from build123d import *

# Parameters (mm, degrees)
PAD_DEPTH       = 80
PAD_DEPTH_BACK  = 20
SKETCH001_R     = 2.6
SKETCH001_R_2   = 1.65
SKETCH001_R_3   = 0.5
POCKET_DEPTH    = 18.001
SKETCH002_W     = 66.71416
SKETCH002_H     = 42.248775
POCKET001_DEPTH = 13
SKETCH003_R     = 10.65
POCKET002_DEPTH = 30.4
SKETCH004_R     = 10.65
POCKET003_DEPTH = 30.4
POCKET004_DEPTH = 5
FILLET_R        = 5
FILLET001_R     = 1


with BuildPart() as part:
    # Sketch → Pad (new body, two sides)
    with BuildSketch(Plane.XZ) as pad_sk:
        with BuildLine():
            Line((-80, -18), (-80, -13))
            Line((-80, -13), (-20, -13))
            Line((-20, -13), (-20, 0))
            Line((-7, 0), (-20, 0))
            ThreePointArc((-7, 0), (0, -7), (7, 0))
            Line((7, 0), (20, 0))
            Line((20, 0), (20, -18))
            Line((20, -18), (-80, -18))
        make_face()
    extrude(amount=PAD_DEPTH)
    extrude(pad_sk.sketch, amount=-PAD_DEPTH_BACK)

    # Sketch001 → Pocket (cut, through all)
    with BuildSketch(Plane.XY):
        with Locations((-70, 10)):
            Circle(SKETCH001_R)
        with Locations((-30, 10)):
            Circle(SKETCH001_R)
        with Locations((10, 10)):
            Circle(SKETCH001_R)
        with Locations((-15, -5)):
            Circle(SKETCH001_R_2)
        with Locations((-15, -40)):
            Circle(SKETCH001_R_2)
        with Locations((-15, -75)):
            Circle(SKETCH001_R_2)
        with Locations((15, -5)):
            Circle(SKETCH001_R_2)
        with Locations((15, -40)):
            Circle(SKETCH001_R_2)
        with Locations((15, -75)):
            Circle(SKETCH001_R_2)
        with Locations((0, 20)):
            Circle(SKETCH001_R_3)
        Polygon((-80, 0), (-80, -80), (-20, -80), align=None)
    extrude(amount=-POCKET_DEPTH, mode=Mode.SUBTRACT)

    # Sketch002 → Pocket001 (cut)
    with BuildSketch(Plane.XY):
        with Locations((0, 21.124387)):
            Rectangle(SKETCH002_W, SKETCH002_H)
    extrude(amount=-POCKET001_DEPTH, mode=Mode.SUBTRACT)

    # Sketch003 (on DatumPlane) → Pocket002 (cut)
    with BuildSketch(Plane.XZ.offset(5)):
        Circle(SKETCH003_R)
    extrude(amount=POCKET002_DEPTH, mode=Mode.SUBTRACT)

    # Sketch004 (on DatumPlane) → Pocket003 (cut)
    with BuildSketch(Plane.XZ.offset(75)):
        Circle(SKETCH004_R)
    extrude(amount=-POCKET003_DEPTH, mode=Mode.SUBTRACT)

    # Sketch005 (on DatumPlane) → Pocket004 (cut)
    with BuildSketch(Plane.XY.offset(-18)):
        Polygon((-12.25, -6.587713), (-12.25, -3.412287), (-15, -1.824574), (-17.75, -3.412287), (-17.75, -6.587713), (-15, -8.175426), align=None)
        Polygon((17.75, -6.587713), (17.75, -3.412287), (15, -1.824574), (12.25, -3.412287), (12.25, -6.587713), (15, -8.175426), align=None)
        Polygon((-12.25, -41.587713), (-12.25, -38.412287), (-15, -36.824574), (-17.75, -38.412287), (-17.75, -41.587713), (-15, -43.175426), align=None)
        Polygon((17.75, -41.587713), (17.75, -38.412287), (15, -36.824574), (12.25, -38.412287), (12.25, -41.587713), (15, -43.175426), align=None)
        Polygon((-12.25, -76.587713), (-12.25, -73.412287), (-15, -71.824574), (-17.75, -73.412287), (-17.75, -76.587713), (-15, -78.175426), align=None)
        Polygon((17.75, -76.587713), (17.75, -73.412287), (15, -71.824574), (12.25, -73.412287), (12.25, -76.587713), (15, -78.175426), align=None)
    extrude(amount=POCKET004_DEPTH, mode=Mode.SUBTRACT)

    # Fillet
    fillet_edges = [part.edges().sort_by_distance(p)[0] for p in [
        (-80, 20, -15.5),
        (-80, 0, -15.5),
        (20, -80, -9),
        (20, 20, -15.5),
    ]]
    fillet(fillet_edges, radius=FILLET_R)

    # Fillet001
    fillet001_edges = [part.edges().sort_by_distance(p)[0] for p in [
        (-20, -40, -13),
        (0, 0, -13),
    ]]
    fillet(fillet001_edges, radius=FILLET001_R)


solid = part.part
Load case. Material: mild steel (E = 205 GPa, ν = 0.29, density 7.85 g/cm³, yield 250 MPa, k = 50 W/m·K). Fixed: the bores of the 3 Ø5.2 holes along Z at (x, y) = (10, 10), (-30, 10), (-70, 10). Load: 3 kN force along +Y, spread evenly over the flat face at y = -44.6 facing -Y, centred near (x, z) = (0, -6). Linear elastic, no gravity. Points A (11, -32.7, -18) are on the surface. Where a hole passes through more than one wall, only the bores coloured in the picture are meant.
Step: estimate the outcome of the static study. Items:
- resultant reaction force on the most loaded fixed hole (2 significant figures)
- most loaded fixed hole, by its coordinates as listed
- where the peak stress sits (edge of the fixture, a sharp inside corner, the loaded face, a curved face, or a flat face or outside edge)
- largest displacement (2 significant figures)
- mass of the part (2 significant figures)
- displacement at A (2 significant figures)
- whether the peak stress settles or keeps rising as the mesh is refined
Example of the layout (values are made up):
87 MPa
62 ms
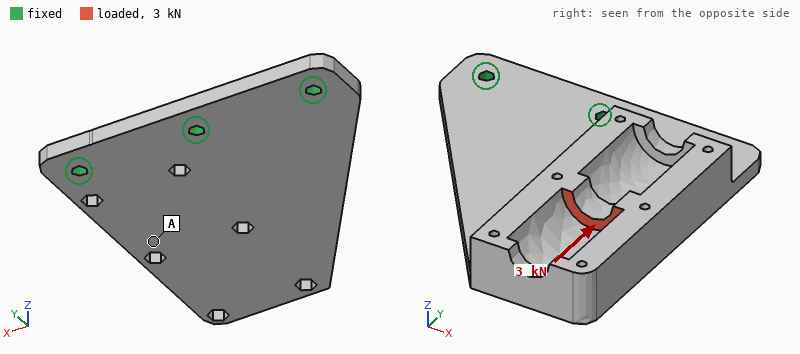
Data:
2.1 kN
(10, 10)
edge of the fixture
0.25 mm
510 g
0.10 mm
keeps rising
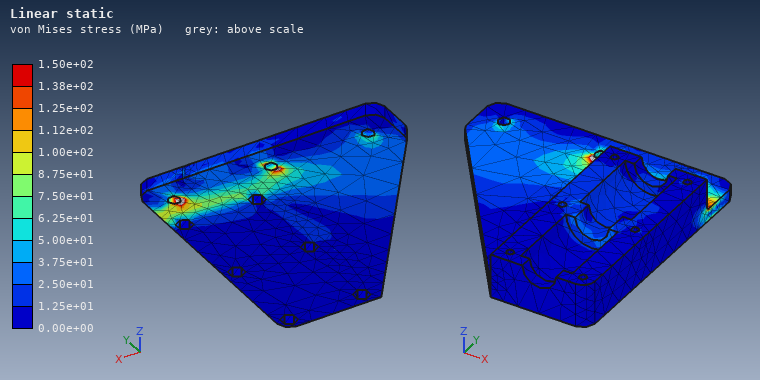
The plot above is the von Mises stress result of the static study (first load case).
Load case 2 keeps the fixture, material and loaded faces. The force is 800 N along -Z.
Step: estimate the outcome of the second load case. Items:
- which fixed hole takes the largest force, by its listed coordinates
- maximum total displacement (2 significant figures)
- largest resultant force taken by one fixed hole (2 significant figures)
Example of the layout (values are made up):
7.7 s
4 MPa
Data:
(10, 10)
0.33 mm
610 N
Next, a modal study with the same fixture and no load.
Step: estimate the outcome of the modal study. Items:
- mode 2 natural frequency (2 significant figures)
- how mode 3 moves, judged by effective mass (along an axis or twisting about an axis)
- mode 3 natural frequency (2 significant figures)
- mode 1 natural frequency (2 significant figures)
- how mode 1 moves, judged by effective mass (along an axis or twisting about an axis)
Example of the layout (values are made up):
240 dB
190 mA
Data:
2700 Hz
along X
4800 Hz
520 Hz
along Z
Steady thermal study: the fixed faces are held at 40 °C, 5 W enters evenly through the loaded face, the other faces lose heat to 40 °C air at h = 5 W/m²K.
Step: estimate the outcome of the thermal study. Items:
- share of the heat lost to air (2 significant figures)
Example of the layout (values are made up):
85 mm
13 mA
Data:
13 %
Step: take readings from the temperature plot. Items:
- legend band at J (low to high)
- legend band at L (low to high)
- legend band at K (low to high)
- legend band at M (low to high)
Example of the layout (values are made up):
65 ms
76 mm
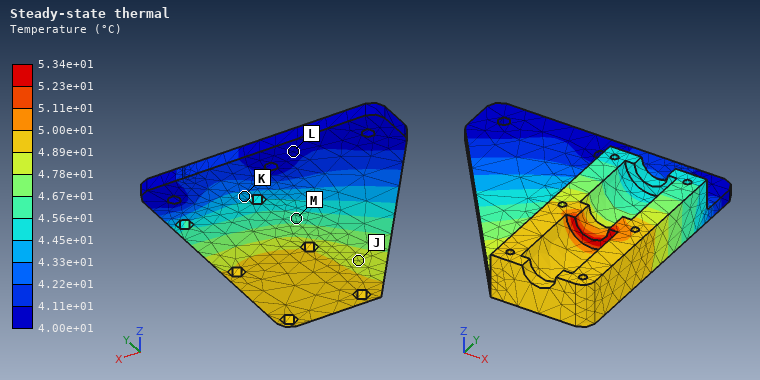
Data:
4.78e+01 to 4.89e+01 °C
4.00e+01 to 4.11e+01 °C
4.33e+01 to 4.45e+01 °C
4.56e+01 to 4.67e+01 °C
